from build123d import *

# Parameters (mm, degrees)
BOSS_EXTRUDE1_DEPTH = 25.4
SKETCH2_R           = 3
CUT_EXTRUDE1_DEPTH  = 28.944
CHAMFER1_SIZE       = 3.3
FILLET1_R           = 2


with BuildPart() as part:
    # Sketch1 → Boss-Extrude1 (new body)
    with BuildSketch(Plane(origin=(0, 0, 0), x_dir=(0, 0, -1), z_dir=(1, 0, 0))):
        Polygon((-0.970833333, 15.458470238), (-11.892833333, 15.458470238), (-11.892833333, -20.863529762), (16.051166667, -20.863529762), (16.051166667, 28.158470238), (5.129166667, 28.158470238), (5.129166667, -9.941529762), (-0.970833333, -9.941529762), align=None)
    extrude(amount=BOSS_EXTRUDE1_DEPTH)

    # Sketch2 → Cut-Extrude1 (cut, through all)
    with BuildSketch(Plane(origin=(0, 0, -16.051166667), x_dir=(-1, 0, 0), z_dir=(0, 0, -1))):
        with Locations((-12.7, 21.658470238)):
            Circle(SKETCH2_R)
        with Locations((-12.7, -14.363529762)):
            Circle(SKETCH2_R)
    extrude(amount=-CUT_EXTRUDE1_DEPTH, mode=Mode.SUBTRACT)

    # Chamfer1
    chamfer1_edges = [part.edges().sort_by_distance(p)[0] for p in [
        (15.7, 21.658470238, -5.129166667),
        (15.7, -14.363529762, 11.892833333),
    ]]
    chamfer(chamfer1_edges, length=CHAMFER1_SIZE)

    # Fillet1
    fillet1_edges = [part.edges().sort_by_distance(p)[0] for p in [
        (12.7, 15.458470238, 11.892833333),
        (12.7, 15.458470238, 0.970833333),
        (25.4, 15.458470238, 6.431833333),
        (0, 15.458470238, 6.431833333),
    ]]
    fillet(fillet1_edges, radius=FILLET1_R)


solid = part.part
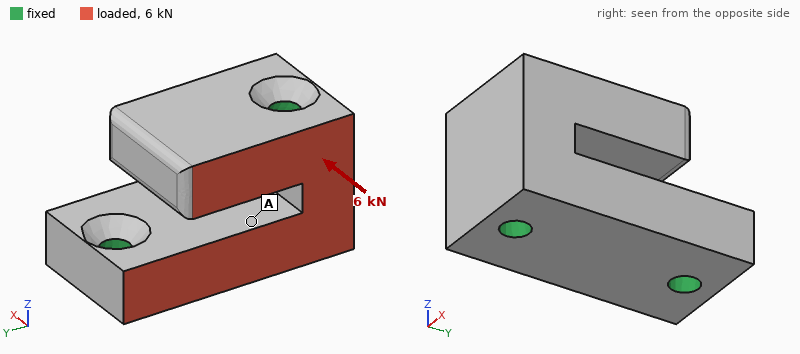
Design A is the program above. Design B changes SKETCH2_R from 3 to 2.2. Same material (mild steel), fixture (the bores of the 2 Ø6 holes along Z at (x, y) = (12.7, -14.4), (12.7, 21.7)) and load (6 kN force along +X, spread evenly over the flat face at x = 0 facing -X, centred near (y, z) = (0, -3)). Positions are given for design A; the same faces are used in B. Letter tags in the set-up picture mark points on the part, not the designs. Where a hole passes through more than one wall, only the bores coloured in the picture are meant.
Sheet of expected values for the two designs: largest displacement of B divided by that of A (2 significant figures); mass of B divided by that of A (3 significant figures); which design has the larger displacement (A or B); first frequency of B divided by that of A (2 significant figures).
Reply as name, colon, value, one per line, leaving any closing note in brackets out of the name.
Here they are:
largest displacement of B divided by that of A: 1.3
mass of B divided by that of A: 1.02
which design has the larger displacement: B
first frequency of B divided by that of A: 0.96
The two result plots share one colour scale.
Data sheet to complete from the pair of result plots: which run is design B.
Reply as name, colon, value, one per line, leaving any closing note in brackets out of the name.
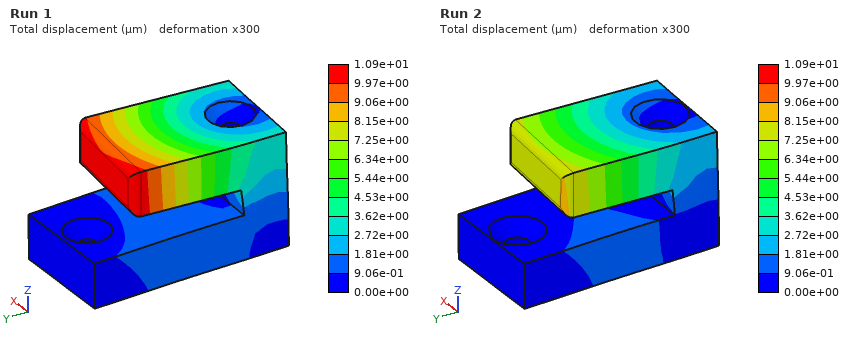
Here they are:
which run is design B: Run 1
